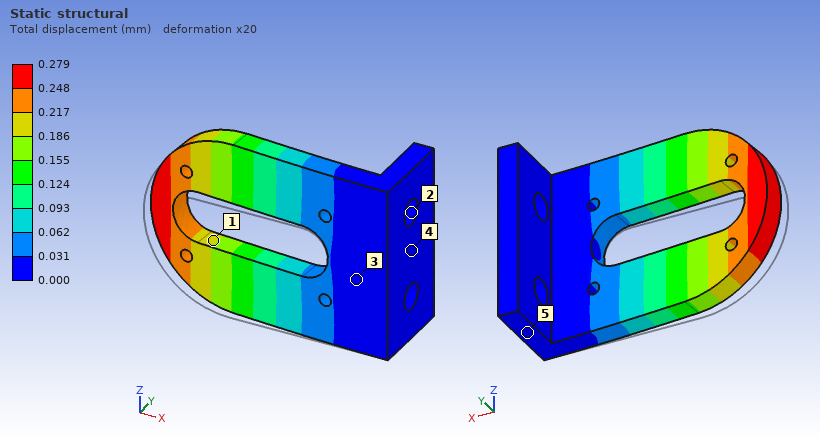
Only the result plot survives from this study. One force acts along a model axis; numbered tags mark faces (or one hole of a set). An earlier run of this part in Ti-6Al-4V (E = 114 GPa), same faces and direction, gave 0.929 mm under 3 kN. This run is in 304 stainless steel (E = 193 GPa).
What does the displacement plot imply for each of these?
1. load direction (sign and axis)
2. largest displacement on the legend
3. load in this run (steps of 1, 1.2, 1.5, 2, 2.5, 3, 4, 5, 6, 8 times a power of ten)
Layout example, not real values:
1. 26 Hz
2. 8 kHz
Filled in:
1. +Y
2. 0.279 mm
3. 1.5 kN
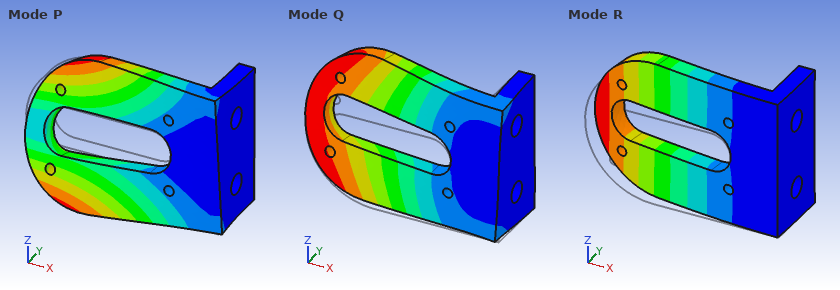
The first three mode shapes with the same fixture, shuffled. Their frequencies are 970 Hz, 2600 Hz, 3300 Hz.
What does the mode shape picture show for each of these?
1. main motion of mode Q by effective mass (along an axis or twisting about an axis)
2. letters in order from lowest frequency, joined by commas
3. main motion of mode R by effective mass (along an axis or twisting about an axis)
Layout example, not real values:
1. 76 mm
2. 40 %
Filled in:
1. along Z
2. R, P, Q
3. along Y
